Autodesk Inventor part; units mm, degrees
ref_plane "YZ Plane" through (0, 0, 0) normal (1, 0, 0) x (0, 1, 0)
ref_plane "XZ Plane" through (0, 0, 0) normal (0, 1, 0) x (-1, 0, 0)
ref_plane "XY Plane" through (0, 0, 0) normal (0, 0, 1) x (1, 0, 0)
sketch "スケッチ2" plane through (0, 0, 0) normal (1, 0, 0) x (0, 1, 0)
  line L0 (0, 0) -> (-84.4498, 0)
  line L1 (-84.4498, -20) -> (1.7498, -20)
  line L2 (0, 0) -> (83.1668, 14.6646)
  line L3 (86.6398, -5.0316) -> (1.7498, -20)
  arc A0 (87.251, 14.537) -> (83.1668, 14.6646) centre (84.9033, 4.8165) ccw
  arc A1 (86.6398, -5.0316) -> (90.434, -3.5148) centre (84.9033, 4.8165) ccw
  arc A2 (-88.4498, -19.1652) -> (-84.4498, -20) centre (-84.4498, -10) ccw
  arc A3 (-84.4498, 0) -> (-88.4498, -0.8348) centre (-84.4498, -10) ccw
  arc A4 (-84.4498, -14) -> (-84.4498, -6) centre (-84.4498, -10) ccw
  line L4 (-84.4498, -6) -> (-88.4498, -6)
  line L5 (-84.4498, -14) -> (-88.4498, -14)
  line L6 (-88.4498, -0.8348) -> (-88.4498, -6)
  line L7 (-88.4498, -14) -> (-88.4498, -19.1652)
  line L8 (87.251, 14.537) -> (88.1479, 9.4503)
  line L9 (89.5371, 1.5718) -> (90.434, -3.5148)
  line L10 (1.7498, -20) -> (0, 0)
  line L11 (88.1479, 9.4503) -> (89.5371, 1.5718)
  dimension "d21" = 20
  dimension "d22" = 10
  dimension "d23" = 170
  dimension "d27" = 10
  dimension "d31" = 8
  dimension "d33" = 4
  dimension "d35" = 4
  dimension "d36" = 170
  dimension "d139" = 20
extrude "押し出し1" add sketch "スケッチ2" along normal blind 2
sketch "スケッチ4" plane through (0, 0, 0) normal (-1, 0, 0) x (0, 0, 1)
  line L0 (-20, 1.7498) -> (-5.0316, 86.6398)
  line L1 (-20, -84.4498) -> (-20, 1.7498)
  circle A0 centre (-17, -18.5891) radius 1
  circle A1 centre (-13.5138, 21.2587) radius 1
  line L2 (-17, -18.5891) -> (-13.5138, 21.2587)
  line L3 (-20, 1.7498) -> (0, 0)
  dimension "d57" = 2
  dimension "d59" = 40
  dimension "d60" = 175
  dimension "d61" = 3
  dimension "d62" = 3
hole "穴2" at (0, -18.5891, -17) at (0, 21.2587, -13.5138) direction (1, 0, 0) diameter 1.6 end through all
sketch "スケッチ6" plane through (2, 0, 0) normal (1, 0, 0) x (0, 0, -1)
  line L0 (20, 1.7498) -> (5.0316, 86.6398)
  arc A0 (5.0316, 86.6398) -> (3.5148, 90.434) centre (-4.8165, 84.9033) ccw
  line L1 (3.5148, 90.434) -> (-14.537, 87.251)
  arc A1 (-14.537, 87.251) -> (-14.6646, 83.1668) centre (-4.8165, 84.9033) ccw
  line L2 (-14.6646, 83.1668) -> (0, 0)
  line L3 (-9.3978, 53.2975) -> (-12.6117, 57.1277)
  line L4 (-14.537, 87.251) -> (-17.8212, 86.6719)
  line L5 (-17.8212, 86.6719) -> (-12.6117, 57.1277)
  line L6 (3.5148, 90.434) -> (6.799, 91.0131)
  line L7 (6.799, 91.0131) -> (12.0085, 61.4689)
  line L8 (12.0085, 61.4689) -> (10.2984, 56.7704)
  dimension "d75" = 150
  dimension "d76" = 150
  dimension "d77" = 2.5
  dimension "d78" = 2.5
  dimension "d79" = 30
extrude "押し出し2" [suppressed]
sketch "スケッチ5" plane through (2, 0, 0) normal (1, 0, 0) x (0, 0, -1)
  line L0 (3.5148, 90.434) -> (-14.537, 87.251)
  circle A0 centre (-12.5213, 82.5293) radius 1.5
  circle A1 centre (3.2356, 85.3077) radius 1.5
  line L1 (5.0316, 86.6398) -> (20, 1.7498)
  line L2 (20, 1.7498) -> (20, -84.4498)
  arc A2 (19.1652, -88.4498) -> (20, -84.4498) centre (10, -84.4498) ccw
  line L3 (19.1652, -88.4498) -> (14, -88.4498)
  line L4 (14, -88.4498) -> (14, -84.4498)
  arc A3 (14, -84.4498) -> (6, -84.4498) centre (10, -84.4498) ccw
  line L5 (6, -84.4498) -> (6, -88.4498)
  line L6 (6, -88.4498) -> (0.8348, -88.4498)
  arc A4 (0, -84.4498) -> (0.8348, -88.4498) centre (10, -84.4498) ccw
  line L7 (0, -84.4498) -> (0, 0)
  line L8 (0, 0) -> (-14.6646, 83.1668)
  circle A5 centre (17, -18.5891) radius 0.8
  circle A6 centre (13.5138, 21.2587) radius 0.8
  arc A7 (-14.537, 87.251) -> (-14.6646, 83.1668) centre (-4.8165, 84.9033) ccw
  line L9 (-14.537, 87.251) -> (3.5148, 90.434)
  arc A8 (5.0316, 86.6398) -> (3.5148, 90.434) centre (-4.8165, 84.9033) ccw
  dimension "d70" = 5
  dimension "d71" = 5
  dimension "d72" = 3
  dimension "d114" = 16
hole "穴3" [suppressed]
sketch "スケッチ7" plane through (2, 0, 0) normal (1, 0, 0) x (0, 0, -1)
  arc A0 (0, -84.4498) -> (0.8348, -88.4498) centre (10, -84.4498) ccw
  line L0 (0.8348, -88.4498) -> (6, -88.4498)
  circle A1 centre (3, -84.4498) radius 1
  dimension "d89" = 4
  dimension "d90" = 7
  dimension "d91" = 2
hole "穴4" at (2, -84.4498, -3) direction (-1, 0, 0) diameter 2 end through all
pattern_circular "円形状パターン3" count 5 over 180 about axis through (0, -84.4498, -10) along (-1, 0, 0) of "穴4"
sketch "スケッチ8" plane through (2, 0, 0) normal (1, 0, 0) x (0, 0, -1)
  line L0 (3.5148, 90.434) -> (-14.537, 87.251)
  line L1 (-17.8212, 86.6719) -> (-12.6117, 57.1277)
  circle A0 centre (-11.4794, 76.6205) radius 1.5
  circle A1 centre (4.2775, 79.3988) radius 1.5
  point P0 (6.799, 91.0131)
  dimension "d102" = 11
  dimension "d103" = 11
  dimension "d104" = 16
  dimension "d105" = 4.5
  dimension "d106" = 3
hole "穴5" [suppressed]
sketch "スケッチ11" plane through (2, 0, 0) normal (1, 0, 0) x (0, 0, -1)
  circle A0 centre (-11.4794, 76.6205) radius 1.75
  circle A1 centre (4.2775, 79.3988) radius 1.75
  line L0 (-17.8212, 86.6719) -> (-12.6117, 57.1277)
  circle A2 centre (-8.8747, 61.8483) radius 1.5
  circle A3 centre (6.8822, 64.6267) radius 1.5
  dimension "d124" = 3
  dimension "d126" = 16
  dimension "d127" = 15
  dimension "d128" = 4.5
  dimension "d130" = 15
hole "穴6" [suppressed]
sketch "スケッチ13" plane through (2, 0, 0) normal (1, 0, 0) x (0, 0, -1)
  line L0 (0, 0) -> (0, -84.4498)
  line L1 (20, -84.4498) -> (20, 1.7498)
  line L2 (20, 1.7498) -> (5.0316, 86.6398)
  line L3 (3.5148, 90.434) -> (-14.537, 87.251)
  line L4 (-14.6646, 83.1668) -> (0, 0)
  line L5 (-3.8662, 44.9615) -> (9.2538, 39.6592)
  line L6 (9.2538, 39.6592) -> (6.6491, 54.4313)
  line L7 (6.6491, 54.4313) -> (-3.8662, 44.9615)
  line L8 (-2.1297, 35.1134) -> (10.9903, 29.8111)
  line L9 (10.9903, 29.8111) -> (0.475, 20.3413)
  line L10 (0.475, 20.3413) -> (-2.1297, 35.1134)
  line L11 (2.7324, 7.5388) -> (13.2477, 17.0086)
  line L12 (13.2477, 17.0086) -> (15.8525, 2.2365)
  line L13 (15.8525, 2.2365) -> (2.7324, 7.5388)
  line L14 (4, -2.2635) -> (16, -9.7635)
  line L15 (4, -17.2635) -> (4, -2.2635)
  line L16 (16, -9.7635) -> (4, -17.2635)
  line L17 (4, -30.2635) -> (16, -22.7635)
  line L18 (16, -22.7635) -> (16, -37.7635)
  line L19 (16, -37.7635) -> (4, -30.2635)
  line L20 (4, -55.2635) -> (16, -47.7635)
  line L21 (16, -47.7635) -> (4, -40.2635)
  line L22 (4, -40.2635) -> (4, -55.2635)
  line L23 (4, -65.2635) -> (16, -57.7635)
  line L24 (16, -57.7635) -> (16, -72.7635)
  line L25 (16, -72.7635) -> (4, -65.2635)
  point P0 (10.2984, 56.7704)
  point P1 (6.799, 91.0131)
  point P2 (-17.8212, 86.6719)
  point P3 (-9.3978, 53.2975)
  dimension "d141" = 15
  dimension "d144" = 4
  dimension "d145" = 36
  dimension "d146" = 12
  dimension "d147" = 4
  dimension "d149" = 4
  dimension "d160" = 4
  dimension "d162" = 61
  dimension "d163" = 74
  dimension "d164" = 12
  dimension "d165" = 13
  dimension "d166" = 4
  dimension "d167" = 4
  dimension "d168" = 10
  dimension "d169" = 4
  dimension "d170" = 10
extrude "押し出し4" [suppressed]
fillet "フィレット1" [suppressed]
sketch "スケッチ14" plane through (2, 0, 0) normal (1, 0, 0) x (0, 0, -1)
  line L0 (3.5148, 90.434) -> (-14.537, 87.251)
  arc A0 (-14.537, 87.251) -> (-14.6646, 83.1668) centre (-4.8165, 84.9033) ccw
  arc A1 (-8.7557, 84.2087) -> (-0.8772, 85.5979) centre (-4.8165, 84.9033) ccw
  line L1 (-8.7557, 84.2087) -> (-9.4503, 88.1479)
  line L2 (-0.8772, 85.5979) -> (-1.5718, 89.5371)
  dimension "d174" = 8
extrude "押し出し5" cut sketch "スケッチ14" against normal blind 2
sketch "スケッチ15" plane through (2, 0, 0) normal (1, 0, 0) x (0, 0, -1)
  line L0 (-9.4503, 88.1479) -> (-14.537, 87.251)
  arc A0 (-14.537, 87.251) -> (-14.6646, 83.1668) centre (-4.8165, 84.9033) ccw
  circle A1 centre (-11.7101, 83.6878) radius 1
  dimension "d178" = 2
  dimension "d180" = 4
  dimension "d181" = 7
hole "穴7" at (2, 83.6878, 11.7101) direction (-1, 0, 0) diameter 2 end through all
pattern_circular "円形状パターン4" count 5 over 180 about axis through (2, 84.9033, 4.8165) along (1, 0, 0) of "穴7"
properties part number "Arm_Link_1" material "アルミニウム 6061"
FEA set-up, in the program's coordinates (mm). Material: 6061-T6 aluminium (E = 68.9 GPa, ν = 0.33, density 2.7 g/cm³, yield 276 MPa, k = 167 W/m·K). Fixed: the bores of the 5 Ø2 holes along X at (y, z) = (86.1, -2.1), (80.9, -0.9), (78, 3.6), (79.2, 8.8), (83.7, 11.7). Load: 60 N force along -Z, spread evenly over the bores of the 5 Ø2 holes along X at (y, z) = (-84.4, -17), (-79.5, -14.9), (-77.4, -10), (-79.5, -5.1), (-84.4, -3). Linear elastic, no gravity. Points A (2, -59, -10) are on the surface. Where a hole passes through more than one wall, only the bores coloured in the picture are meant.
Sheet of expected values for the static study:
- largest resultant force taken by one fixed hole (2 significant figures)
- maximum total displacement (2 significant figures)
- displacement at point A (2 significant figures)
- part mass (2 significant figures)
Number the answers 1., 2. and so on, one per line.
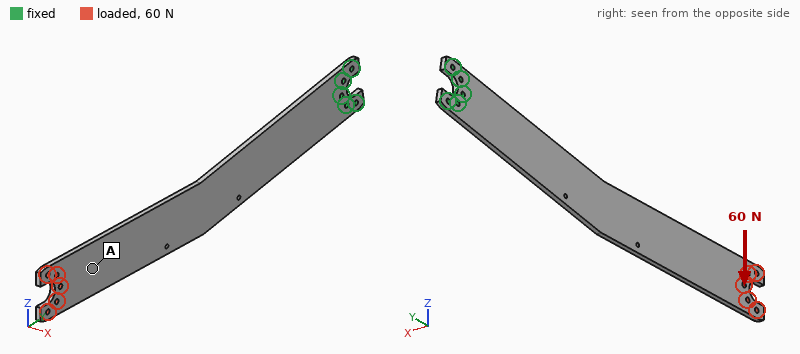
1. 500 N
2. 1.0 mm
3. 0.78 mm
4. 18 g
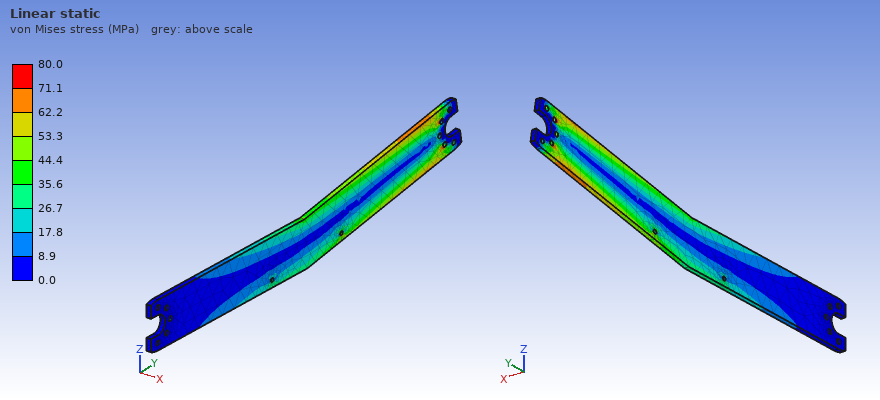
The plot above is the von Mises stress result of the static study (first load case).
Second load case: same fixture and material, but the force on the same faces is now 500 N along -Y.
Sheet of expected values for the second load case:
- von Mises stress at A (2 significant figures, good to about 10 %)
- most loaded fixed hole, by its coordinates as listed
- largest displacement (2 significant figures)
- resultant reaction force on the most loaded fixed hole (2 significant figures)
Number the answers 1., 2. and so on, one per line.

1. 12 MPa
2. (80.9, -0.9)
3. 0.48 mm
4. 480 N
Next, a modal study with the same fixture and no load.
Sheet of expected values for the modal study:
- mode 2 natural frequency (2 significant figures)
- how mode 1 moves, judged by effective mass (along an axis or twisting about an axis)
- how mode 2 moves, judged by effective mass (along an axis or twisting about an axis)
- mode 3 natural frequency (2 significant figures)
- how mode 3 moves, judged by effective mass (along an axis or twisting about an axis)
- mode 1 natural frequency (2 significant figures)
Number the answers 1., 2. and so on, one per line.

1. 370 Hz
2. along X
3. along X
4. 570 Hz
5. along Z
6. 61 Hz
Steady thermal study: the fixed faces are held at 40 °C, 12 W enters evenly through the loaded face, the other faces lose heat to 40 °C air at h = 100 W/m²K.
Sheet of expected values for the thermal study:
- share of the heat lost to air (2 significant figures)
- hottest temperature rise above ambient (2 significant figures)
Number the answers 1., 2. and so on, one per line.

1. 97 %
2. 64 K
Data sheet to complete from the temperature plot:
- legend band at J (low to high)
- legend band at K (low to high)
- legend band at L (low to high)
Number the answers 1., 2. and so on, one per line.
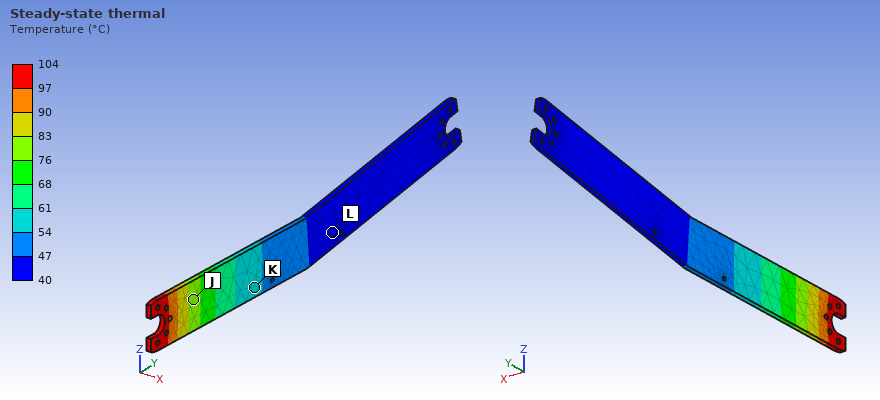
1. 76 to 83 °C
2. 54 to 61 °C
3. 40 to 47 °C
